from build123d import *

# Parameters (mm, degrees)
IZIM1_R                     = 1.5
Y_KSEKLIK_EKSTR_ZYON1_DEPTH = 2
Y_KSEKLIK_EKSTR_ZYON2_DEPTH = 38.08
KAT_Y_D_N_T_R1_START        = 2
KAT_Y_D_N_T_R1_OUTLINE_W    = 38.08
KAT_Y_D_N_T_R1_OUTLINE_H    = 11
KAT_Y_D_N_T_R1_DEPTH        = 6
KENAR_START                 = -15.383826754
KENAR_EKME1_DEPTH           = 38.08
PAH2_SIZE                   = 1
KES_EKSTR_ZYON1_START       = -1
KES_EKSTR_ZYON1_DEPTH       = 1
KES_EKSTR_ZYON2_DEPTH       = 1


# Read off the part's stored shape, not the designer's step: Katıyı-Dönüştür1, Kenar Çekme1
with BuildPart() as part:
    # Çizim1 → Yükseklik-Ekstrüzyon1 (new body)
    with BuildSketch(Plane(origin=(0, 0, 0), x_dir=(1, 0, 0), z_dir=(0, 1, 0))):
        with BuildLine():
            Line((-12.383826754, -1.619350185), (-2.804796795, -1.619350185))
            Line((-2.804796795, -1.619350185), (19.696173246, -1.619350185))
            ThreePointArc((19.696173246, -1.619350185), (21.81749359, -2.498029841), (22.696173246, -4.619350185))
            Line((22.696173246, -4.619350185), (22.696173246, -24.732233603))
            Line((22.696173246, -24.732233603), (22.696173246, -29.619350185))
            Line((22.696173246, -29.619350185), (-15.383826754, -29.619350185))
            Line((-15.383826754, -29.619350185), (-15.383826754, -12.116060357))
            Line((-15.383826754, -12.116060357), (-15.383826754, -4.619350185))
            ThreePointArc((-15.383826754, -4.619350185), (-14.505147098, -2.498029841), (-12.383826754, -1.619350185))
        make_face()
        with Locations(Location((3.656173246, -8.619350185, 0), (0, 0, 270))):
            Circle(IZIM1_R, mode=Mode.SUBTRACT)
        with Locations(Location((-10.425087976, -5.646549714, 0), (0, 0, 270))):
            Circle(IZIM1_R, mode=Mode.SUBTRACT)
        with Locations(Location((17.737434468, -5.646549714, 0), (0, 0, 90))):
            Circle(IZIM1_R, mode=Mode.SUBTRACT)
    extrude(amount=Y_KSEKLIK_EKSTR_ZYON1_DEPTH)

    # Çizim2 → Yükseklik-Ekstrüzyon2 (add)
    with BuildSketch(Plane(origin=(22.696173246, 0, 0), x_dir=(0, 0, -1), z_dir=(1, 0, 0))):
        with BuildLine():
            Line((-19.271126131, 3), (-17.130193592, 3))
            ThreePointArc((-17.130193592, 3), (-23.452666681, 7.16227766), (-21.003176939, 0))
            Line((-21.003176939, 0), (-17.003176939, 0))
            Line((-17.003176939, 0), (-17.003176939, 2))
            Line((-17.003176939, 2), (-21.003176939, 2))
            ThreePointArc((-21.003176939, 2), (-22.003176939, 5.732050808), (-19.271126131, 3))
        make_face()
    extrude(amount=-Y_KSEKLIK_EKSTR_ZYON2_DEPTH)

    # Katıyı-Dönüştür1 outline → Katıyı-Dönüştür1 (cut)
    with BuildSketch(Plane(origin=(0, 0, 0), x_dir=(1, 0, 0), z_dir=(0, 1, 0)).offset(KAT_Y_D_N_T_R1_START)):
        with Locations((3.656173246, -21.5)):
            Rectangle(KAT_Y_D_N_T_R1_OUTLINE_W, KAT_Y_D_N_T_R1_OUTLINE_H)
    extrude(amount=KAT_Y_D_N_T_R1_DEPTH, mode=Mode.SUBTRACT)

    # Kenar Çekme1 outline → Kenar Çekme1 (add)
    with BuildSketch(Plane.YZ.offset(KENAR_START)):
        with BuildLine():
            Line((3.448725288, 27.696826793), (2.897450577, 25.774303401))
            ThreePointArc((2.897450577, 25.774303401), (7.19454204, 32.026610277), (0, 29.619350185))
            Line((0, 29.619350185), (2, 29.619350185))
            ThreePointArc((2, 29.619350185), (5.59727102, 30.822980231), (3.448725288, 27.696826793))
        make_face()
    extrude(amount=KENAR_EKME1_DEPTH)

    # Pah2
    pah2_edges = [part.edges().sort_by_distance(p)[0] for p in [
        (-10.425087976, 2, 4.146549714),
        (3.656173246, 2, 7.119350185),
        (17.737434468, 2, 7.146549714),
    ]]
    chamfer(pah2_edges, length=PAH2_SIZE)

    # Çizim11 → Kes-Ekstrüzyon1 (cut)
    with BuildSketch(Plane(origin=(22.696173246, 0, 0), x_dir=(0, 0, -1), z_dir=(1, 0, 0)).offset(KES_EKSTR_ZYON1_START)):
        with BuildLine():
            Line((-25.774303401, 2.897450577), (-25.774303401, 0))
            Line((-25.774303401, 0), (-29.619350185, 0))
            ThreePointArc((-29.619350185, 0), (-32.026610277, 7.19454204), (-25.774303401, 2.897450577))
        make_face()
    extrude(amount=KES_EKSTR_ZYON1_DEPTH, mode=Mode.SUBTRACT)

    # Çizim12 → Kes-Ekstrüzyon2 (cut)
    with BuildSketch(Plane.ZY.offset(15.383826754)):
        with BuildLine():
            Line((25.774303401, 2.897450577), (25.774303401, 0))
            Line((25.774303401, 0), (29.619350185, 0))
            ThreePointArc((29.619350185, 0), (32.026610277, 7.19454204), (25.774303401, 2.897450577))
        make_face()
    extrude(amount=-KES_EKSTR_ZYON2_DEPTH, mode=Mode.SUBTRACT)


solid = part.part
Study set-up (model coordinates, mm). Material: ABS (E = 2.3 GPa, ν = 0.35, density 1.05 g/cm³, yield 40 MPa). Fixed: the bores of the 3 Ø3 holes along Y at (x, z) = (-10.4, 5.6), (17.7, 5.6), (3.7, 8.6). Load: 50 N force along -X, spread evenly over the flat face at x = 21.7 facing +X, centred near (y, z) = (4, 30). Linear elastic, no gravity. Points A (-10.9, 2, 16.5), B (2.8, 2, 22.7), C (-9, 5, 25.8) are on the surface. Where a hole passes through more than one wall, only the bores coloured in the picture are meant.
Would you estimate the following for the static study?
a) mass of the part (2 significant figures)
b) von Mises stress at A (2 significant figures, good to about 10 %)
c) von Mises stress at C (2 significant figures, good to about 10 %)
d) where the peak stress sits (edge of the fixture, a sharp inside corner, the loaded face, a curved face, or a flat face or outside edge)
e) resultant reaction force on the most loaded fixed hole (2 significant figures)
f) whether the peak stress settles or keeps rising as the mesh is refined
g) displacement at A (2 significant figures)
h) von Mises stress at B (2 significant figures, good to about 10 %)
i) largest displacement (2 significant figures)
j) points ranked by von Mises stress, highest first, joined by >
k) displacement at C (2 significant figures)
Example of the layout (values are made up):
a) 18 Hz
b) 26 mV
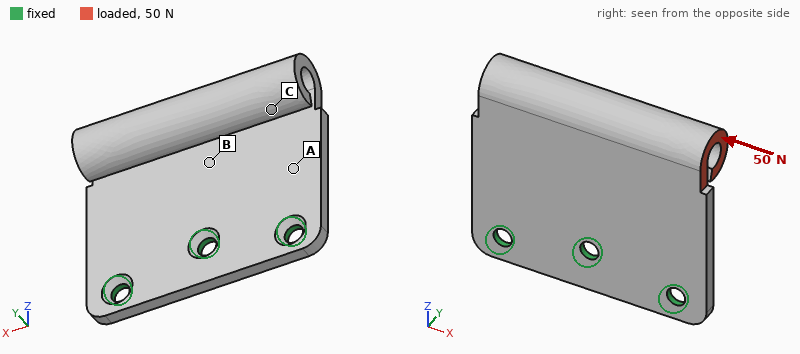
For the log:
a) 3.3 g
b) 3.8 MPa
c) 1.2 MPa
d) edge of the fixture
e) 41 N
f) keeps rising
g) 0.11 mm
h) 5.4 MPa
i) 0.54 mm
j) B > A > C
k) 0.33 mm
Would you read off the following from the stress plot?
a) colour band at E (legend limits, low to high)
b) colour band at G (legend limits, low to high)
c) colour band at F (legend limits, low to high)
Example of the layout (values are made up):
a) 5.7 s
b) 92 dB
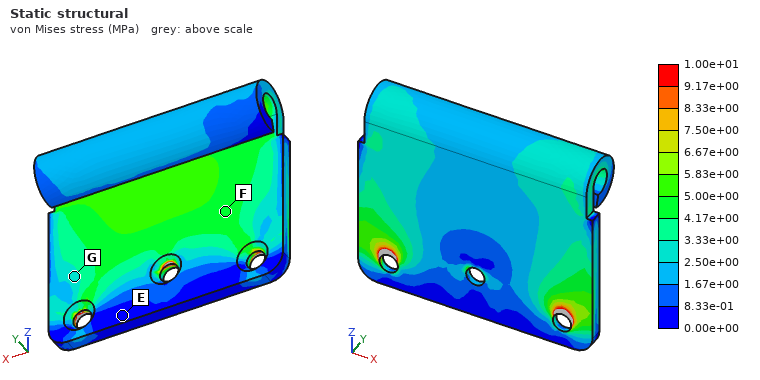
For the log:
a) 0.00e+00 to 8.33e-01 MPa
b) 2.50e+00 to 3.33e+00 MPa
c) 4.17e+00 to 5.00e+00 MPa
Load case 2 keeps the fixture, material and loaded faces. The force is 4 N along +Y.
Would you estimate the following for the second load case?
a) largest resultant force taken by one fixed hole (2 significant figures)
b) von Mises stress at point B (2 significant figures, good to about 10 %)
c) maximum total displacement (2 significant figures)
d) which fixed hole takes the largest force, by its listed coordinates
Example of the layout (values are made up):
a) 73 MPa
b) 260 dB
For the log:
a) 5.3 N
b) 2.0 MPa
c) 0.60 mm
d) (3.7, 8.6)
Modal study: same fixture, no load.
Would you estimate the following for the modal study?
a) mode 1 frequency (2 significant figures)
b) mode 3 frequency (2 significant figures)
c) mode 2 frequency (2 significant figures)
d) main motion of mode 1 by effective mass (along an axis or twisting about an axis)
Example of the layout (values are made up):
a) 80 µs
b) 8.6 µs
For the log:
a) 450 Hz
b) 2300 Hz
c) 860 Hz
d) along Y
